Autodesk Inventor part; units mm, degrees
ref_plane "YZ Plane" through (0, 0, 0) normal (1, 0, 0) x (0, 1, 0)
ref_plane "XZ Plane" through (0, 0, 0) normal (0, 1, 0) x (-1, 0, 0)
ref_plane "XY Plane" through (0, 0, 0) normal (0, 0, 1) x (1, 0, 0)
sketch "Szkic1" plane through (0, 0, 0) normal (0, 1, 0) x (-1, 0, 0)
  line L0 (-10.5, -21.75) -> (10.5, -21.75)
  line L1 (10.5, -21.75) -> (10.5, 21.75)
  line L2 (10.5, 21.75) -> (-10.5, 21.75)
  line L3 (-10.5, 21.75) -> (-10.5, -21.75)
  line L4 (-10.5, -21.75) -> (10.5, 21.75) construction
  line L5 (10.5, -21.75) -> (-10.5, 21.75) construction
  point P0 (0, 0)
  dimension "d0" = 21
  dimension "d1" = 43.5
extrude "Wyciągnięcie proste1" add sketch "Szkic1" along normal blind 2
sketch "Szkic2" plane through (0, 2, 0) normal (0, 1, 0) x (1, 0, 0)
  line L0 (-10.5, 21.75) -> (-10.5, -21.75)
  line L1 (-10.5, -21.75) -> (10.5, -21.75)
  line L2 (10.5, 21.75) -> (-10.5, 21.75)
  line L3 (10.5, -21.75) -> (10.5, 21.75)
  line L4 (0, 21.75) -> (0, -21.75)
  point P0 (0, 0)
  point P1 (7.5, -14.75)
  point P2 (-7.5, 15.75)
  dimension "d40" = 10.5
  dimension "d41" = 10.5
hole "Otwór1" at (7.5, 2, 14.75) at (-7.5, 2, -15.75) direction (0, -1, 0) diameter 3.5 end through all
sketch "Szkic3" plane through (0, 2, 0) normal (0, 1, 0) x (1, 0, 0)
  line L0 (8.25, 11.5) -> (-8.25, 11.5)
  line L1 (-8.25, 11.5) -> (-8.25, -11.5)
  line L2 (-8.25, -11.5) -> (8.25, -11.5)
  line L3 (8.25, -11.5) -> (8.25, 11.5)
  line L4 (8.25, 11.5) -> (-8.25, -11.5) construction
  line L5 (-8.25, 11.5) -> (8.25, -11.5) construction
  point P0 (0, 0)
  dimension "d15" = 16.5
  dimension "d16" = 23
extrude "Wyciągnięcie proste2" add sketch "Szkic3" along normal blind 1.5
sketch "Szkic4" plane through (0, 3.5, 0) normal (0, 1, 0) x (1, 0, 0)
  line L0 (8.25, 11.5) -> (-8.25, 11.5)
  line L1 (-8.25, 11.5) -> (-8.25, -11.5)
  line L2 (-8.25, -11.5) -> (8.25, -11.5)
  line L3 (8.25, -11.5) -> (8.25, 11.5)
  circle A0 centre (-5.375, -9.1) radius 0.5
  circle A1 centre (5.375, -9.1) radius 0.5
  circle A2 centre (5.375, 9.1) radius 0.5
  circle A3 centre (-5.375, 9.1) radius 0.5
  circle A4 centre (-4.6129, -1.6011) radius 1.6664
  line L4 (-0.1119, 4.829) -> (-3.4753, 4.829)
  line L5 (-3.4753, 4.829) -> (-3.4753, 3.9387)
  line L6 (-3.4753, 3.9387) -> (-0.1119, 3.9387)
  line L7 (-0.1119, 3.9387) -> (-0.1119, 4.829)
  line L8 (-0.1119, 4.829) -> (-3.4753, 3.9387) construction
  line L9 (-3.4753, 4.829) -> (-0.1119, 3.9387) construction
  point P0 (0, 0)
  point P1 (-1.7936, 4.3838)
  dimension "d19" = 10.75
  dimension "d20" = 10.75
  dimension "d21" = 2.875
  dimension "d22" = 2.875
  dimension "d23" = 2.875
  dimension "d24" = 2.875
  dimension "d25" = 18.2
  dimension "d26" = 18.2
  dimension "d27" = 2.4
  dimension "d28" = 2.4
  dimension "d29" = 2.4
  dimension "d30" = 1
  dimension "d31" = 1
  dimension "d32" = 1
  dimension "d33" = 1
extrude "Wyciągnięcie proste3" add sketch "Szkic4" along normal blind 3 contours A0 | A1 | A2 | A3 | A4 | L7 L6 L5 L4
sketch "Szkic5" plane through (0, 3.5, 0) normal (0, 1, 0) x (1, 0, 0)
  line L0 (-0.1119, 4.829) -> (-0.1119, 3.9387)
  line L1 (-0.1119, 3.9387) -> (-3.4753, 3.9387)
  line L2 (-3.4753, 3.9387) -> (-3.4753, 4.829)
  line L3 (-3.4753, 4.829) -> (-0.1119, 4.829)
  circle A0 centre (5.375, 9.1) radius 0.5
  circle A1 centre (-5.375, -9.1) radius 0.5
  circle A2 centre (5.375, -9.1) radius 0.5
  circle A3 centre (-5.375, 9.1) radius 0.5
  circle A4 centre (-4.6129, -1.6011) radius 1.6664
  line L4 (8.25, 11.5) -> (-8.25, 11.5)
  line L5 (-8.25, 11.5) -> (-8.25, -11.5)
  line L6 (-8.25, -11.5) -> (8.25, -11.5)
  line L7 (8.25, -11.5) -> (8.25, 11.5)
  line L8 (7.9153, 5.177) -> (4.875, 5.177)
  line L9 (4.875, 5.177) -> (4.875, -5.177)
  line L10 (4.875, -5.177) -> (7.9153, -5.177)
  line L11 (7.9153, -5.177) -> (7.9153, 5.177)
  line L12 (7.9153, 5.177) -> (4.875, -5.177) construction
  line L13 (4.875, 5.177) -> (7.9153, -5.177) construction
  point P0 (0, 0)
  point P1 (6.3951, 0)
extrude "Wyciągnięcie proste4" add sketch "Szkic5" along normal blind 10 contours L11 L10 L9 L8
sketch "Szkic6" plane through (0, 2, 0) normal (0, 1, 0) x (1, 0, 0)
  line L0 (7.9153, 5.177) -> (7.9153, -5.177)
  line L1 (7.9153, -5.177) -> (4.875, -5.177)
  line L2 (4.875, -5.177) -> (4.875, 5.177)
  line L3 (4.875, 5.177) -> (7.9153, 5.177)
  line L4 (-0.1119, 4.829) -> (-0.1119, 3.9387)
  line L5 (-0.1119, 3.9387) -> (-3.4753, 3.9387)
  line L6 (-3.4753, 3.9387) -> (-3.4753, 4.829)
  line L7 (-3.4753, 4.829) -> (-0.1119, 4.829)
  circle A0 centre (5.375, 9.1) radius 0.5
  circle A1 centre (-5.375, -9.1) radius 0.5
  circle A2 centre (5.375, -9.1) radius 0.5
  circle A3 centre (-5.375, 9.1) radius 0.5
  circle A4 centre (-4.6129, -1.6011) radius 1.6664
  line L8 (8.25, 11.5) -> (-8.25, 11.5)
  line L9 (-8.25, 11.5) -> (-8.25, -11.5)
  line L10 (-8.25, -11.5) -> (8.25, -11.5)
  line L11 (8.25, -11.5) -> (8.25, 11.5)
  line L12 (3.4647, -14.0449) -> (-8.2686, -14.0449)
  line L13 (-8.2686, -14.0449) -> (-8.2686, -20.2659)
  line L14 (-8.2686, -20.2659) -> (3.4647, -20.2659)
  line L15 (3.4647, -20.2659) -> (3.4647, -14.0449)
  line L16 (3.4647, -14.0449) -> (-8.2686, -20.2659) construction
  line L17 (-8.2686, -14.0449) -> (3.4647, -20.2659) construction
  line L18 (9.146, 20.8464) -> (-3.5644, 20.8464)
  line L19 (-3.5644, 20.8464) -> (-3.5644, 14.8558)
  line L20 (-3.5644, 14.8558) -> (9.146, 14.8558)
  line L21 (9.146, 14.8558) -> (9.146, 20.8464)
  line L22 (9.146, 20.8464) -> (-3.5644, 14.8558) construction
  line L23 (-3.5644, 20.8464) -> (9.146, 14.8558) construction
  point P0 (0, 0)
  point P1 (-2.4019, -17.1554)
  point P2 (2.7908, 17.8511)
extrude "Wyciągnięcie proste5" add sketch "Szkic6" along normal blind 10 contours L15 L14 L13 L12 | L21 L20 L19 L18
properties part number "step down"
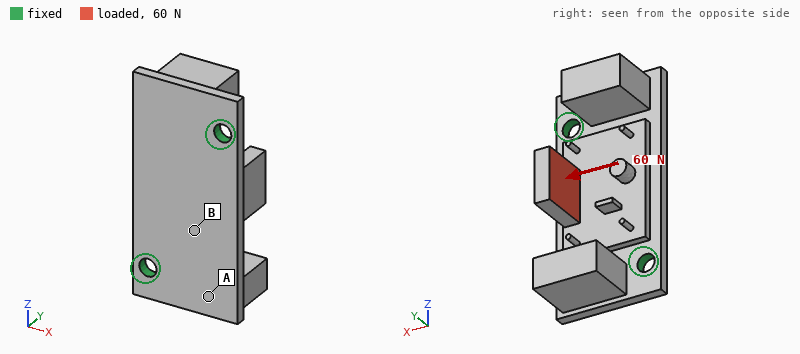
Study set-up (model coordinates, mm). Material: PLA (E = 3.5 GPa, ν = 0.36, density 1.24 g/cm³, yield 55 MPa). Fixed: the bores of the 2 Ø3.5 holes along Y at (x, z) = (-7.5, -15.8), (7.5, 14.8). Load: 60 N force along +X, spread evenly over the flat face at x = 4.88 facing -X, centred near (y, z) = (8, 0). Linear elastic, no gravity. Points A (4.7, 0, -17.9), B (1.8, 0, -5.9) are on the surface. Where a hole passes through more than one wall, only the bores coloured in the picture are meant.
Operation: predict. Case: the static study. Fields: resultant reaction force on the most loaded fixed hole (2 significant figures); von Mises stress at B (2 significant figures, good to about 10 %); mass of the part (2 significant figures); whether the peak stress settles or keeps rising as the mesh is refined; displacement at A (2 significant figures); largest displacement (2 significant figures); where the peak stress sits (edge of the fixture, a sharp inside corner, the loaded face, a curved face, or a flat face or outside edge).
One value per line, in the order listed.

32 N
4.8 MPa
5.2 g
keeps rising
0.15 mm
0.47 mm
edge of the fixture
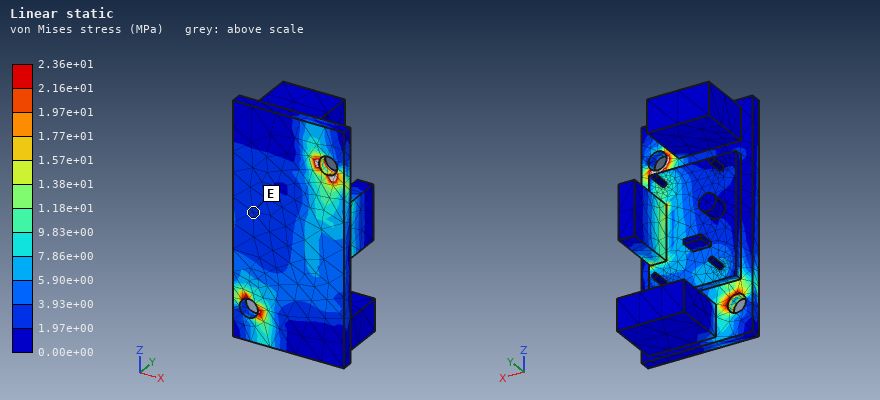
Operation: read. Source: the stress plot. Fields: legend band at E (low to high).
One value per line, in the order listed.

1.97e+00 to 3.93e+00 MPa
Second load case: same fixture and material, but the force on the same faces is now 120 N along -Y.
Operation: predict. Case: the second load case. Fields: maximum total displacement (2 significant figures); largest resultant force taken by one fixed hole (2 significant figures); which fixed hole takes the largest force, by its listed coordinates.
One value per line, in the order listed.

0.54 mm
100 N
(7.5, 14.8)
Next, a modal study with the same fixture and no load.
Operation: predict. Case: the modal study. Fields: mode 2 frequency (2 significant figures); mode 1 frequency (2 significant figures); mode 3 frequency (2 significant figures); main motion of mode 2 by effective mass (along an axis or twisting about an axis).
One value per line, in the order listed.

1800 Hz
1200 Hz
2700 Hz
along Y
